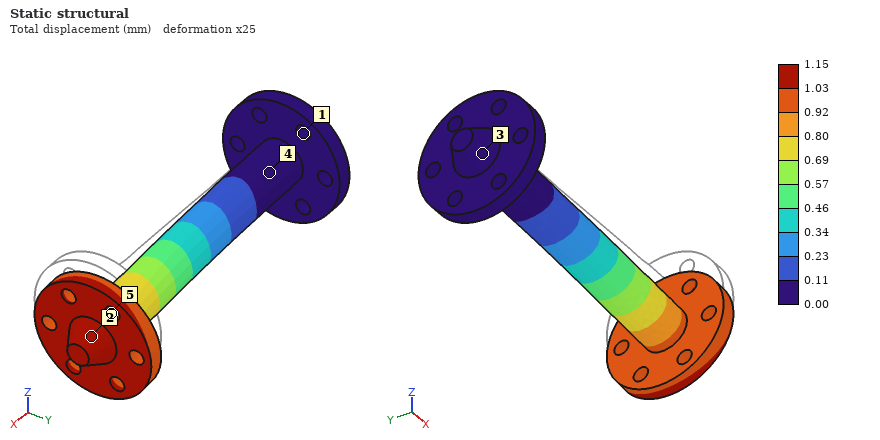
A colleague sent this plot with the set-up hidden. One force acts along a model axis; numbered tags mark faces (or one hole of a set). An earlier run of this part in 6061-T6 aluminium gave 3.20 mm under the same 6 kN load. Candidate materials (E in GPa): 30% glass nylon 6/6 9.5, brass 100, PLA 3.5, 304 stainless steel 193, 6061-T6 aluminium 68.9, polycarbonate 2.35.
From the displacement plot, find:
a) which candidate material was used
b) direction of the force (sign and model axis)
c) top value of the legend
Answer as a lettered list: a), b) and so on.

a) 304 stainless steel
b) -Z
c) 1.15 mm
